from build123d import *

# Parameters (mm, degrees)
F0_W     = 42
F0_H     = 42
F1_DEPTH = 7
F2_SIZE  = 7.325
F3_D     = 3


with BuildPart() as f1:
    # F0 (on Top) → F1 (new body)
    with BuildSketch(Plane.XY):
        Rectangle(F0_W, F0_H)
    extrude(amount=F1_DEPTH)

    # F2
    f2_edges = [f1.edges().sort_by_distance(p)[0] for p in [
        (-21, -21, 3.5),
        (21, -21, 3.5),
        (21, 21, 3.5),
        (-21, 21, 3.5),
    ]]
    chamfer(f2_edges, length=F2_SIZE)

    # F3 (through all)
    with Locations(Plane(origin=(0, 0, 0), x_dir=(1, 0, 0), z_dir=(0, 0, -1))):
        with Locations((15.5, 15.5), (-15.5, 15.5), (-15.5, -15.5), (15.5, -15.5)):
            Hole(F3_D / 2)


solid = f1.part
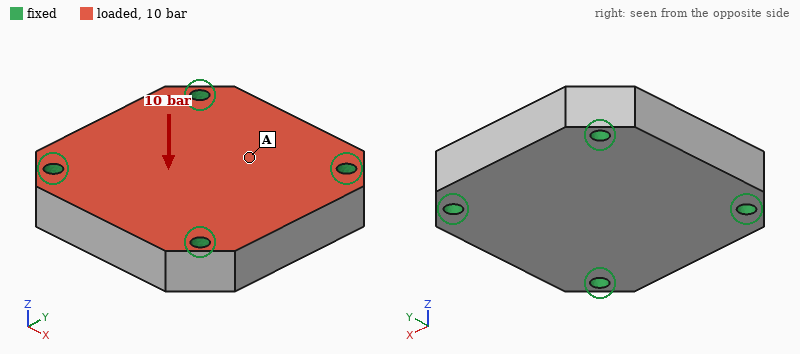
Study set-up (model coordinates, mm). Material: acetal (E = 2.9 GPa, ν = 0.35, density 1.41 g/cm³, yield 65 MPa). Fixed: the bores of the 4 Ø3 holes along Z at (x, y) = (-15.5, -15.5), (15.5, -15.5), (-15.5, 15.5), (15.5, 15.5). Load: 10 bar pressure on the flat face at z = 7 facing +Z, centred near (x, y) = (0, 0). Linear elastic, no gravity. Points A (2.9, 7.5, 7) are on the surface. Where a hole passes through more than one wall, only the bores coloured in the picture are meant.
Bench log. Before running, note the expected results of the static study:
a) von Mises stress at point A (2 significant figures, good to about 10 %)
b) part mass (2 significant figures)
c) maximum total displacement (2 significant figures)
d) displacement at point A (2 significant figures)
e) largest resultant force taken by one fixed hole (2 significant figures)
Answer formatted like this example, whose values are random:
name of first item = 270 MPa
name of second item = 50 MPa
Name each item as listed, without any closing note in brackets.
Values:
von Mises stress at point A = 4.9 MPa
part mass = 16 g
maximum total displacement = 0.11 mm
displacement at point A = 0.092 mm
largest resultant force taken by one fixed hole = 410 N
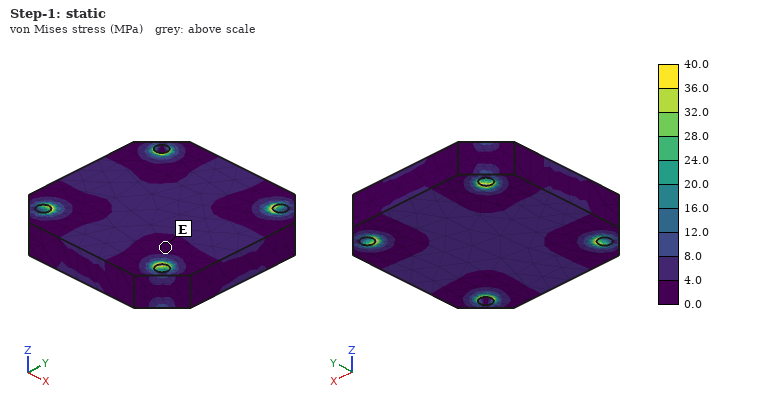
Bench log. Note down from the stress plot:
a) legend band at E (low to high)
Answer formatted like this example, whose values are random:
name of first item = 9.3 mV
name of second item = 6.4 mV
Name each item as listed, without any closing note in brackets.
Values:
legend band at E = 0.0 to 4.0 MPa
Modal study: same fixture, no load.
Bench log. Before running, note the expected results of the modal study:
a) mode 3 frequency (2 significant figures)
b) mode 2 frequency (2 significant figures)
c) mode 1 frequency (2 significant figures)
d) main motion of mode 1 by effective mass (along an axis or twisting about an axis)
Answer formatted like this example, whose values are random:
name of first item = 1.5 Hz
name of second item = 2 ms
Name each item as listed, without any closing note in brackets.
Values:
mode 3 frequency = 8600 Hz
mode 2 frequency = 8600 Hz
mode 1 frequency = 5800 Hz
main motion of mode 1 by effective mass = along Z
